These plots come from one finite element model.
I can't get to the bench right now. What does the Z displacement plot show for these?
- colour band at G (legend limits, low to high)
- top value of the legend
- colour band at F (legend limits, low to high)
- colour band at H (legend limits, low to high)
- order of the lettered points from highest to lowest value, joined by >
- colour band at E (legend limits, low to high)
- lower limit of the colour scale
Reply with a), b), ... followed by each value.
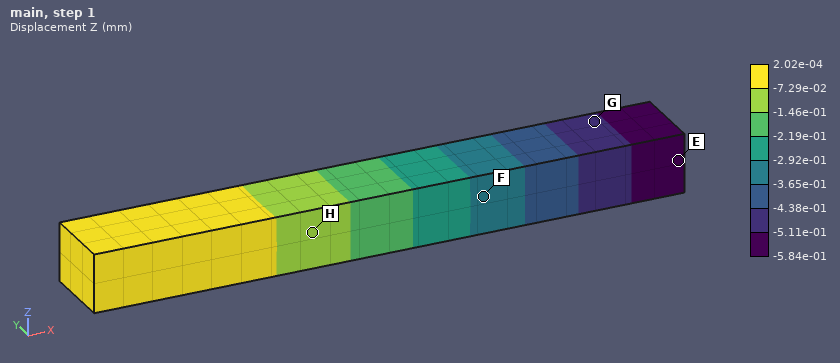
a) -5.11e-01 to -4.38e-01 mm
b) 2.02e-04 mm
c) -3.65e-01 to -2.92e-01 mm
d) -1.46e-01 to -7.29e-02 mm
e) H > F > G > E
f) -5.84e-01 to -5.11e-01 mm
g) -5.84e-01 mm
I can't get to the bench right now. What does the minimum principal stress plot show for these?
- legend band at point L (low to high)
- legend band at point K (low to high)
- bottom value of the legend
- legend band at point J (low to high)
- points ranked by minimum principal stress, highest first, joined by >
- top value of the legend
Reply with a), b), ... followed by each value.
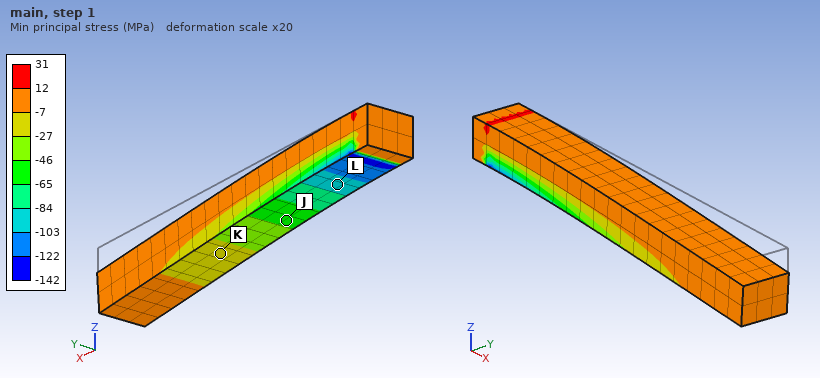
a) -103 to -84 MPa
b) -27 to -7 MPa
c) -142 MPa
d) -65 to -46 MPa
e) K > J > L
f) 31 MPa
